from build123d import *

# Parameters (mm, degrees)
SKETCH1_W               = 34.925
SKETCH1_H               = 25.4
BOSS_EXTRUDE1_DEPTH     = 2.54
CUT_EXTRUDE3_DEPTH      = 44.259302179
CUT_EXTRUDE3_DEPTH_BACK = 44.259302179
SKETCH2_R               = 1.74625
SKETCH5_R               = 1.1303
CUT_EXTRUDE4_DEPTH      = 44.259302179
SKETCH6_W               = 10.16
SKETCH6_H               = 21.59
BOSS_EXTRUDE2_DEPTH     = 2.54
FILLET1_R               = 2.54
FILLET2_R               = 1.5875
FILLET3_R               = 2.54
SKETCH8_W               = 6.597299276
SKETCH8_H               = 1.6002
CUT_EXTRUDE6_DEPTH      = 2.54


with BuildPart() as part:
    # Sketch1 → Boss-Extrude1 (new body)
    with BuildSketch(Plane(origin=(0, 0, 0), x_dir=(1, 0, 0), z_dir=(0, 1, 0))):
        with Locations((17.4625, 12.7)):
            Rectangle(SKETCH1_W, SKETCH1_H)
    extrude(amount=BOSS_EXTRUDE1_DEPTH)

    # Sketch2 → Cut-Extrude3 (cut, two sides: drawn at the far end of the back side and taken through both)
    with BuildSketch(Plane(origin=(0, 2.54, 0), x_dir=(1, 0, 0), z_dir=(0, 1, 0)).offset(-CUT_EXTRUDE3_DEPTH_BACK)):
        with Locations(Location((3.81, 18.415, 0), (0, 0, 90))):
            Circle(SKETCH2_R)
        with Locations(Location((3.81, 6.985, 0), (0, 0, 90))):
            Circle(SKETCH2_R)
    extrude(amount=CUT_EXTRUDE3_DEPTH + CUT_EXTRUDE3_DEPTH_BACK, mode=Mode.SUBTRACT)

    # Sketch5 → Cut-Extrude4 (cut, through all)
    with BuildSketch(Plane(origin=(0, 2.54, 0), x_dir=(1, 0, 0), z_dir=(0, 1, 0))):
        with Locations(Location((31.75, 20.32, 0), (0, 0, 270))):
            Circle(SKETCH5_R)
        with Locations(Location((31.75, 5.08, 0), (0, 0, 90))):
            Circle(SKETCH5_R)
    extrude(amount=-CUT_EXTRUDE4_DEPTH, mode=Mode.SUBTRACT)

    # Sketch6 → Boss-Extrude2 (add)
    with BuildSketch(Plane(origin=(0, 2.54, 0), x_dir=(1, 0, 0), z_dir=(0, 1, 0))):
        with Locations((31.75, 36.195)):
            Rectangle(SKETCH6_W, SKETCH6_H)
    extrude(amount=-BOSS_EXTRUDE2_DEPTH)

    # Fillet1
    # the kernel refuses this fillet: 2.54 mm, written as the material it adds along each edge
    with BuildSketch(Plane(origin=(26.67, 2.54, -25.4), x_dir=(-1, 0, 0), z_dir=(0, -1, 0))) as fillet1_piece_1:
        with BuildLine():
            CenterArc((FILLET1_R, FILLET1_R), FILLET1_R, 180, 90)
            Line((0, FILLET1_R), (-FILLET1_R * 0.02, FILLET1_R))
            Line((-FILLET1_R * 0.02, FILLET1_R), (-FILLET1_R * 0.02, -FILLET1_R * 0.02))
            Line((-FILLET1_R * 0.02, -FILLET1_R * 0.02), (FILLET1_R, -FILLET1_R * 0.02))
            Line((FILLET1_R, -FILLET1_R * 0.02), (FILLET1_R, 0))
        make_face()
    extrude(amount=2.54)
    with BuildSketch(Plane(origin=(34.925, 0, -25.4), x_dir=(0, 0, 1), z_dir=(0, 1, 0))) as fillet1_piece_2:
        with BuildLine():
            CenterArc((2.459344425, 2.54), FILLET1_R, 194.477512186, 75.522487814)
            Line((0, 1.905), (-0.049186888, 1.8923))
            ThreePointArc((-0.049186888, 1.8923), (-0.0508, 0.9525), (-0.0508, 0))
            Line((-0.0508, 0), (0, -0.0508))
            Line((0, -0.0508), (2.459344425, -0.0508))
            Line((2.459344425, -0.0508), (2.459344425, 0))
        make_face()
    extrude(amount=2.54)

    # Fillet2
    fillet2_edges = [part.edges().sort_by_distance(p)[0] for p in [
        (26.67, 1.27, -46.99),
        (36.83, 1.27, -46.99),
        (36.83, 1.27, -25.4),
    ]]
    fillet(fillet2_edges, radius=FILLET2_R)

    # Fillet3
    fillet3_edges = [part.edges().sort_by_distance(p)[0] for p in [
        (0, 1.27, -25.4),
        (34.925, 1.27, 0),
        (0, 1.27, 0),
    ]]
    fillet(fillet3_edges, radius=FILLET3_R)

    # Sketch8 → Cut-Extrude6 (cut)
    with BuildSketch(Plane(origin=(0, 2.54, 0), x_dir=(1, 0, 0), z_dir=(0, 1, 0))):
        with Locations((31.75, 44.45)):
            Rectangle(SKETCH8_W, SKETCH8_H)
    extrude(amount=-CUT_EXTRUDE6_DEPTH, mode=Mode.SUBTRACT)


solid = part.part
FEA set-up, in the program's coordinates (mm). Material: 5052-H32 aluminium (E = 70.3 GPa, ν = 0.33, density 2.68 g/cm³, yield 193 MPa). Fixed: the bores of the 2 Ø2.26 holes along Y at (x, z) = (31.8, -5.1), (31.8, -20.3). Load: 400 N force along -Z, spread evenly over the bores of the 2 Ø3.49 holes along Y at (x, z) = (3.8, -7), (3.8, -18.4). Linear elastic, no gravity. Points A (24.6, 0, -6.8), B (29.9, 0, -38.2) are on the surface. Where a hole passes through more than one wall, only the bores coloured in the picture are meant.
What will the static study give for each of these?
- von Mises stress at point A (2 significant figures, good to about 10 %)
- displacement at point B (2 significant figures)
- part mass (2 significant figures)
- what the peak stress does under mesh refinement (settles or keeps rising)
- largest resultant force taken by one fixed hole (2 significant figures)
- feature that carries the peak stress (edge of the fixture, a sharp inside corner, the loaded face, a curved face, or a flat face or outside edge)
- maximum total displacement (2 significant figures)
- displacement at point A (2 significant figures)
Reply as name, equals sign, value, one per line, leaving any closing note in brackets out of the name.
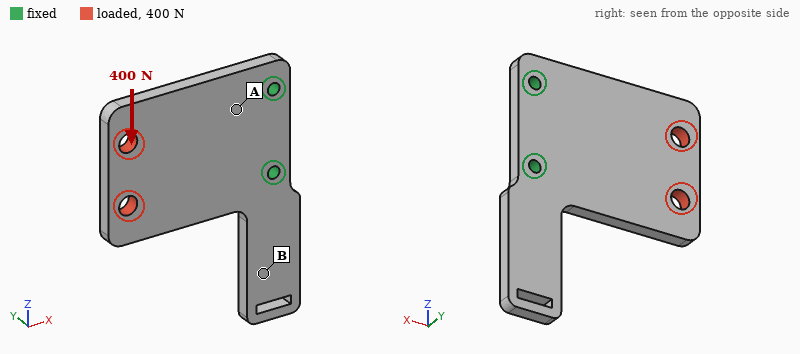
von Mises stress at point A = 24 MPa
displacement at point B = 15 µm
part mass = 7.3 g
what the peak stress does under mesh refinement = keeps rising
largest resultant force taken by one fixed hole = 700 N
feature that carries the peak stress = edge of the fixture
maximum total displacement = 29 µm
displacement at point A = 4.9 µm
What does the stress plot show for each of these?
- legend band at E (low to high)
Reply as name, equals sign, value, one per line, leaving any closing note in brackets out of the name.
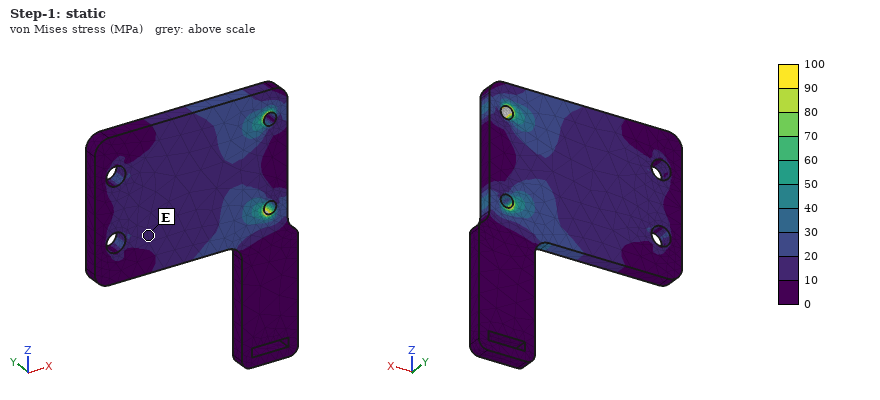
legend band at E = 10 to 20 MPa
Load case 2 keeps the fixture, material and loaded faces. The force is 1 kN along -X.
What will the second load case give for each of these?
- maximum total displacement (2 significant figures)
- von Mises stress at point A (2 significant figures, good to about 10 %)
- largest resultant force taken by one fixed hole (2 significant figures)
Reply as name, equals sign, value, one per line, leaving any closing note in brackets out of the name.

maximum total displacement = 9.2 µm
von Mises stress at point A = 18 MPa
largest resultant force taken by one fixed hole = 500 N
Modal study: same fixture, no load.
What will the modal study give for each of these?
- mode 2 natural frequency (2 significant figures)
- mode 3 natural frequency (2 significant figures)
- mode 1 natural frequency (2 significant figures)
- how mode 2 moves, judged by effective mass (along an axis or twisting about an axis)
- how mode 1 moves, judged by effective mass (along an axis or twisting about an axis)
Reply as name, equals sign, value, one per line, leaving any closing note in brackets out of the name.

mode 2 natural frequency = 3200 Hz
mode 3 natural frequency = 6000 Hz
mode 1 natural frequency = 2100 Hz
how mode 2 moves, judged by effective mass = along Y
how mode 1 moves, judged by effective mass = along Y
